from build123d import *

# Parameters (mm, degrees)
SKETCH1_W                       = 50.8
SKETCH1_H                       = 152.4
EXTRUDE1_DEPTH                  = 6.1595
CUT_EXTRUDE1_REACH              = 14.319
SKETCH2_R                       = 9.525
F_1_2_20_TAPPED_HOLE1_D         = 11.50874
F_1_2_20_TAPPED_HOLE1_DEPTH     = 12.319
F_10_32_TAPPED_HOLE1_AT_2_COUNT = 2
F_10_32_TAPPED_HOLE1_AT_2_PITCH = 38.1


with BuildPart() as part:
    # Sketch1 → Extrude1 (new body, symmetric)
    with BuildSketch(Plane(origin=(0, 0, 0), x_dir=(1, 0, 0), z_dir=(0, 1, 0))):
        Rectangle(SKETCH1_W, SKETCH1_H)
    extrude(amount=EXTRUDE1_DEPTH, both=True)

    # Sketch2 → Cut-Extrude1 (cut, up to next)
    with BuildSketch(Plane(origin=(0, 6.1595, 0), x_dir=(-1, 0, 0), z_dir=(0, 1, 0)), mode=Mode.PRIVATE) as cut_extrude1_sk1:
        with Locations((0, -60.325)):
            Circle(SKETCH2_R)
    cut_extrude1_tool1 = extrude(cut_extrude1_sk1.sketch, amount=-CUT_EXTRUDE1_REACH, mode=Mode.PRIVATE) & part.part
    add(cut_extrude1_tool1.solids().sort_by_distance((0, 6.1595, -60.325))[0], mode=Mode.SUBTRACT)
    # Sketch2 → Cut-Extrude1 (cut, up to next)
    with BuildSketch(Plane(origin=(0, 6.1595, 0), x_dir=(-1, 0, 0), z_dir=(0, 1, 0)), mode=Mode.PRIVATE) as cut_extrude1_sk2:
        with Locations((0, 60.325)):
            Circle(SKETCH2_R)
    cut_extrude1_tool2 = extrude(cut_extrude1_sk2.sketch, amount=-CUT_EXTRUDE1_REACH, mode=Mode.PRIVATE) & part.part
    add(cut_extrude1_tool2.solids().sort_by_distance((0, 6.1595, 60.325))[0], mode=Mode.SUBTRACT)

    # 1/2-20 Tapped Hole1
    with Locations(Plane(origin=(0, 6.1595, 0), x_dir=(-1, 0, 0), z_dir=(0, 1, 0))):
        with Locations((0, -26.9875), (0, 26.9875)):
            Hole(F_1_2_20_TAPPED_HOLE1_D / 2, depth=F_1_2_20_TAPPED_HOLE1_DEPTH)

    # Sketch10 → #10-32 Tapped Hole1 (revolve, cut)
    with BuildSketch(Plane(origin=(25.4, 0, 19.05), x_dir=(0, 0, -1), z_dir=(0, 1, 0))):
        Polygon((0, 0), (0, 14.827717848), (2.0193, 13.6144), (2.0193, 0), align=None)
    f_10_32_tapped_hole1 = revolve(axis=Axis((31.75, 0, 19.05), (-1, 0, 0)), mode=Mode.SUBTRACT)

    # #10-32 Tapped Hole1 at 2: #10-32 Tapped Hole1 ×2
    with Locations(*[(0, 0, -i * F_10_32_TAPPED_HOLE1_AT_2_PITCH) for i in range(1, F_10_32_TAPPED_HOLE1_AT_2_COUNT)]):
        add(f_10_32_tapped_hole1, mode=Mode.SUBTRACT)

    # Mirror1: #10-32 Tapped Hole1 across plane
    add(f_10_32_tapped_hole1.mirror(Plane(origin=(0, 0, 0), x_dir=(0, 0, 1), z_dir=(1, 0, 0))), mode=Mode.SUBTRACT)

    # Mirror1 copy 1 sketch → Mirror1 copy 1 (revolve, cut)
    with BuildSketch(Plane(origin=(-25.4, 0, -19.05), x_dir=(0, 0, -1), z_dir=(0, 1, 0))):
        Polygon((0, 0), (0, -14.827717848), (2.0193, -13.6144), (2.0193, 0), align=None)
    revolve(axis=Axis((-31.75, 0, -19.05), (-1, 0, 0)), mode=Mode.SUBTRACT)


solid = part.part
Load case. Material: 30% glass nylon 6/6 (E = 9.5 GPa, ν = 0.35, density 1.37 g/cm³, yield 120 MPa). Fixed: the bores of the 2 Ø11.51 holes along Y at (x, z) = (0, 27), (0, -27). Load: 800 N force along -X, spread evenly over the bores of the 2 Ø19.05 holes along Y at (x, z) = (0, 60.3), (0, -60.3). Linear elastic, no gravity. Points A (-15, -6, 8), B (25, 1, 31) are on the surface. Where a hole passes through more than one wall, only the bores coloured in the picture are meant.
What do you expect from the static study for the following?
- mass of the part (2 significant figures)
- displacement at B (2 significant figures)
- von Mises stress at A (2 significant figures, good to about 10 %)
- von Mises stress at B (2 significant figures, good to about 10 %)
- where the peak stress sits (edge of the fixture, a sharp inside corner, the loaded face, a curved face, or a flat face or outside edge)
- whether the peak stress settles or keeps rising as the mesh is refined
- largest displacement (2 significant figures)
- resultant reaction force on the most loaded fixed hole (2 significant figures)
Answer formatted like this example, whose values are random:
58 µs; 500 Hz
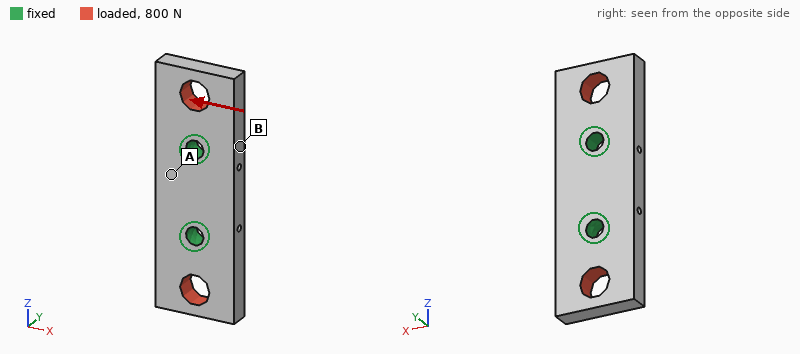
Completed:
120 g; 7.3 µm; 0.95 MPa; 2.2 MPa; edge of the fixture; keeps rising; 32 µm; 400 N
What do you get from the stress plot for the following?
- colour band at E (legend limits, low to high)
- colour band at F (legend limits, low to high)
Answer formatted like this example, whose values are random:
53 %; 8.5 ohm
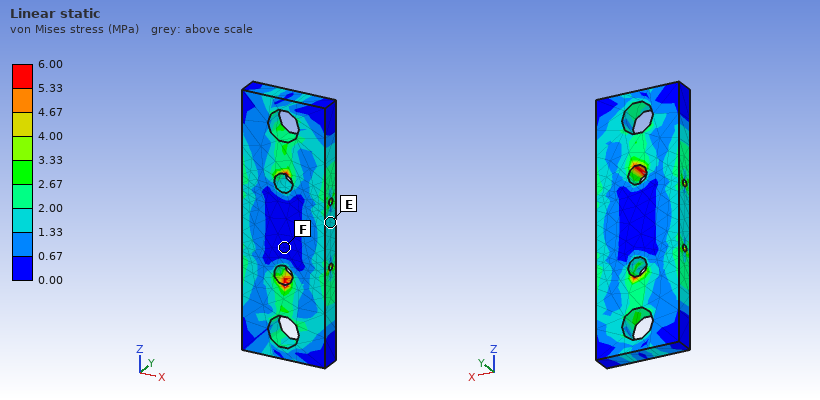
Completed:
1.33 to 2.00 MPa; 0.00 to 0.67 MPa
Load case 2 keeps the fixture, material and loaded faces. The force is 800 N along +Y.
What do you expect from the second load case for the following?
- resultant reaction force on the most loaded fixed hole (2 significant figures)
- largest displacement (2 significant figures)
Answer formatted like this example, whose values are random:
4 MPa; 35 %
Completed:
400 N; 0.13 mm
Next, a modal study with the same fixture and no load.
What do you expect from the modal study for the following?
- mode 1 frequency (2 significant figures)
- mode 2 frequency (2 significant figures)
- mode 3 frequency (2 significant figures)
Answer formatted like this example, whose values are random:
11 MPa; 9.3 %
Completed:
2200 Hz; 2300 Hz; 3400 Hz
